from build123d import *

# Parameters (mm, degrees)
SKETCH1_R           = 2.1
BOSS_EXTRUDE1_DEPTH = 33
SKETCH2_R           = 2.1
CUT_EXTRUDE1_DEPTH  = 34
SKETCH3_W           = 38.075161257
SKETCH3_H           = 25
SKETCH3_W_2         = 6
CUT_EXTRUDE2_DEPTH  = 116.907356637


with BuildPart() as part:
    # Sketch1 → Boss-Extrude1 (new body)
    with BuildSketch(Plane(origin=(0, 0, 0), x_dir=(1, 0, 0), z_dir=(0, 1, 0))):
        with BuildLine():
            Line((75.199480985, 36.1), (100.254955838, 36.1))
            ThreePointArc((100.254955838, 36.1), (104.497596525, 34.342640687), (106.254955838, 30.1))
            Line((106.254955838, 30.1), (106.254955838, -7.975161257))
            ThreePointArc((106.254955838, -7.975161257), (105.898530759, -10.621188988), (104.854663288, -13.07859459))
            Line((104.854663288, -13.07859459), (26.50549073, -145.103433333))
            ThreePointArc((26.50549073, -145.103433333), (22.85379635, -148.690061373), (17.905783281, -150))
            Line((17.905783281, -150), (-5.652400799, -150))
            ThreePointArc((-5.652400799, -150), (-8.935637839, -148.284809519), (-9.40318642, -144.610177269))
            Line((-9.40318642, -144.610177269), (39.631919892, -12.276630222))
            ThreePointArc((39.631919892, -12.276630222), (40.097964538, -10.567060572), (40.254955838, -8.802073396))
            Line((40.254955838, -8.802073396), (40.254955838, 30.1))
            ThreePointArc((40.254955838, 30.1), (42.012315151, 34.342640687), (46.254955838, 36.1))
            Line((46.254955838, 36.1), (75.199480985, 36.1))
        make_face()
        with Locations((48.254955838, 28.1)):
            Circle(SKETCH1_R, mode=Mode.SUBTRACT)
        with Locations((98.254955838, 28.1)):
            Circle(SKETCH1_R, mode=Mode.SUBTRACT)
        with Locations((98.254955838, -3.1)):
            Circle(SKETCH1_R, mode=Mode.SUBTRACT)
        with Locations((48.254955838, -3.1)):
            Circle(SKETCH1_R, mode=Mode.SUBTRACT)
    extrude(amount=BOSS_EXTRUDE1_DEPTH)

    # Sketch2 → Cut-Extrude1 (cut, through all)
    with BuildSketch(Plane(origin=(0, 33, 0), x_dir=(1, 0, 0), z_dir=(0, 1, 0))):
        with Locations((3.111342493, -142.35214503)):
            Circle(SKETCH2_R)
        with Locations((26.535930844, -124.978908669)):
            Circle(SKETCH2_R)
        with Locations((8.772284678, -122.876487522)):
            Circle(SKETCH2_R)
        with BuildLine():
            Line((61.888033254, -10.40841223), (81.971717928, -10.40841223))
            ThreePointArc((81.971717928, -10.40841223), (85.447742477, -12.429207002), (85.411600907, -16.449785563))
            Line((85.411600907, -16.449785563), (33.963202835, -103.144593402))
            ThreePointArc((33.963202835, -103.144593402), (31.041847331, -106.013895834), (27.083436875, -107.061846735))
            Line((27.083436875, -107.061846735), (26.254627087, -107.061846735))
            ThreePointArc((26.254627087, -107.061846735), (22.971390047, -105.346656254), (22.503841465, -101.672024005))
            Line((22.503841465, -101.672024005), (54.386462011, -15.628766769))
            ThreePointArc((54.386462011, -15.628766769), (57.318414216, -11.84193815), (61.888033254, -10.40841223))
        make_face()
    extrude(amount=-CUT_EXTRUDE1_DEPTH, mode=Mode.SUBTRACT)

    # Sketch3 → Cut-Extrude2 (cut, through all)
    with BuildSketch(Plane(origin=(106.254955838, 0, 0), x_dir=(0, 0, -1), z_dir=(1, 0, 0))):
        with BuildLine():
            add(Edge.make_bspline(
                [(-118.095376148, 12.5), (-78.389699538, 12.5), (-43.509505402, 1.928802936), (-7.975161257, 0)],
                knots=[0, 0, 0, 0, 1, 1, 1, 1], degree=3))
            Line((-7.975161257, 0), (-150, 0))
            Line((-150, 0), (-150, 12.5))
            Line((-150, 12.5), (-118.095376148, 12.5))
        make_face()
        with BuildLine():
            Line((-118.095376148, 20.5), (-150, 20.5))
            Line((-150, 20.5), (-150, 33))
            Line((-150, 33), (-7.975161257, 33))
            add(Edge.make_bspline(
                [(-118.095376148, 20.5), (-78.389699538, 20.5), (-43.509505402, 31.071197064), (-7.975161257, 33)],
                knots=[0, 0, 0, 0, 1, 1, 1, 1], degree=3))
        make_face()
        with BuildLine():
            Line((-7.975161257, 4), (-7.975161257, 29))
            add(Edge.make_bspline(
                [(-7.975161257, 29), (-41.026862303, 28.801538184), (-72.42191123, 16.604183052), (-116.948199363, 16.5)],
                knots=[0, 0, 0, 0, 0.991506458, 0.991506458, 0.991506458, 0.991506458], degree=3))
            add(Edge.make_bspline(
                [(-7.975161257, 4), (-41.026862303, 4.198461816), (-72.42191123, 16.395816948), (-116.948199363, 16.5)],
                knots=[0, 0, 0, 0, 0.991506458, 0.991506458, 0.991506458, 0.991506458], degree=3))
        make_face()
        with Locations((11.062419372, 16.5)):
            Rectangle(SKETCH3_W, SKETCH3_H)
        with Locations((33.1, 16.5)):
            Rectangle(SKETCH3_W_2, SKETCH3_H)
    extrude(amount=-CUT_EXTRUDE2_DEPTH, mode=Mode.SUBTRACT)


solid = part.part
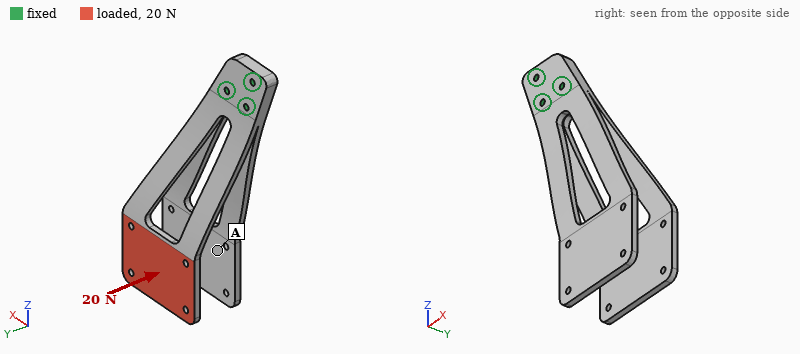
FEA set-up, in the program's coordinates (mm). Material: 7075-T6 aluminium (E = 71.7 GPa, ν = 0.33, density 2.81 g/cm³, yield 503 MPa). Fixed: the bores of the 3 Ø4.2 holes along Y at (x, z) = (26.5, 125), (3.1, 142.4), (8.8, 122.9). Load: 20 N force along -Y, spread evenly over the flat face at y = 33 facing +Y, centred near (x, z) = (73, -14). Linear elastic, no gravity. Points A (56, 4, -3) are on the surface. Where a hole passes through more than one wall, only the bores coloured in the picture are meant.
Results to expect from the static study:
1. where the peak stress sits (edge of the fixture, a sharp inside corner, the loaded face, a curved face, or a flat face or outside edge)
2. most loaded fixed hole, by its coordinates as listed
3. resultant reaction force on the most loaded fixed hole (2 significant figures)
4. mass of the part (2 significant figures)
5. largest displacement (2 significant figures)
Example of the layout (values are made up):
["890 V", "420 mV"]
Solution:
["a curved face", "(26.5, 125)", "45 N", "170 g", "2.2 mm"]
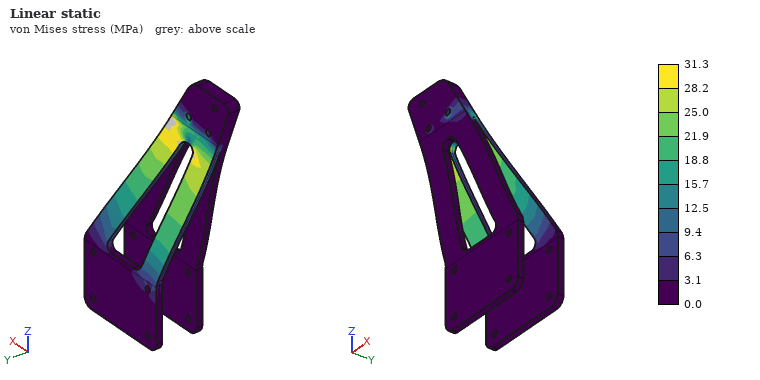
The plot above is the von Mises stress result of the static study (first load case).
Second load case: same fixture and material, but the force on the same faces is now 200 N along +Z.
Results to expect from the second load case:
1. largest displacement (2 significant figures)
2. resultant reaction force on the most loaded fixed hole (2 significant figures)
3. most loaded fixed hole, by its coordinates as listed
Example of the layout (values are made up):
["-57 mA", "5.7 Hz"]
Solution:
["2.6 mm", "530 N", "(26.5, 125)"]
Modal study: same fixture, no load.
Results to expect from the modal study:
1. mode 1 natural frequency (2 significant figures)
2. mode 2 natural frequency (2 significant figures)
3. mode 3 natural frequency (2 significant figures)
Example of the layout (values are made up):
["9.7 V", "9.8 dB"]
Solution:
["89 Hz", "90 Hz", "410 Hz"]
